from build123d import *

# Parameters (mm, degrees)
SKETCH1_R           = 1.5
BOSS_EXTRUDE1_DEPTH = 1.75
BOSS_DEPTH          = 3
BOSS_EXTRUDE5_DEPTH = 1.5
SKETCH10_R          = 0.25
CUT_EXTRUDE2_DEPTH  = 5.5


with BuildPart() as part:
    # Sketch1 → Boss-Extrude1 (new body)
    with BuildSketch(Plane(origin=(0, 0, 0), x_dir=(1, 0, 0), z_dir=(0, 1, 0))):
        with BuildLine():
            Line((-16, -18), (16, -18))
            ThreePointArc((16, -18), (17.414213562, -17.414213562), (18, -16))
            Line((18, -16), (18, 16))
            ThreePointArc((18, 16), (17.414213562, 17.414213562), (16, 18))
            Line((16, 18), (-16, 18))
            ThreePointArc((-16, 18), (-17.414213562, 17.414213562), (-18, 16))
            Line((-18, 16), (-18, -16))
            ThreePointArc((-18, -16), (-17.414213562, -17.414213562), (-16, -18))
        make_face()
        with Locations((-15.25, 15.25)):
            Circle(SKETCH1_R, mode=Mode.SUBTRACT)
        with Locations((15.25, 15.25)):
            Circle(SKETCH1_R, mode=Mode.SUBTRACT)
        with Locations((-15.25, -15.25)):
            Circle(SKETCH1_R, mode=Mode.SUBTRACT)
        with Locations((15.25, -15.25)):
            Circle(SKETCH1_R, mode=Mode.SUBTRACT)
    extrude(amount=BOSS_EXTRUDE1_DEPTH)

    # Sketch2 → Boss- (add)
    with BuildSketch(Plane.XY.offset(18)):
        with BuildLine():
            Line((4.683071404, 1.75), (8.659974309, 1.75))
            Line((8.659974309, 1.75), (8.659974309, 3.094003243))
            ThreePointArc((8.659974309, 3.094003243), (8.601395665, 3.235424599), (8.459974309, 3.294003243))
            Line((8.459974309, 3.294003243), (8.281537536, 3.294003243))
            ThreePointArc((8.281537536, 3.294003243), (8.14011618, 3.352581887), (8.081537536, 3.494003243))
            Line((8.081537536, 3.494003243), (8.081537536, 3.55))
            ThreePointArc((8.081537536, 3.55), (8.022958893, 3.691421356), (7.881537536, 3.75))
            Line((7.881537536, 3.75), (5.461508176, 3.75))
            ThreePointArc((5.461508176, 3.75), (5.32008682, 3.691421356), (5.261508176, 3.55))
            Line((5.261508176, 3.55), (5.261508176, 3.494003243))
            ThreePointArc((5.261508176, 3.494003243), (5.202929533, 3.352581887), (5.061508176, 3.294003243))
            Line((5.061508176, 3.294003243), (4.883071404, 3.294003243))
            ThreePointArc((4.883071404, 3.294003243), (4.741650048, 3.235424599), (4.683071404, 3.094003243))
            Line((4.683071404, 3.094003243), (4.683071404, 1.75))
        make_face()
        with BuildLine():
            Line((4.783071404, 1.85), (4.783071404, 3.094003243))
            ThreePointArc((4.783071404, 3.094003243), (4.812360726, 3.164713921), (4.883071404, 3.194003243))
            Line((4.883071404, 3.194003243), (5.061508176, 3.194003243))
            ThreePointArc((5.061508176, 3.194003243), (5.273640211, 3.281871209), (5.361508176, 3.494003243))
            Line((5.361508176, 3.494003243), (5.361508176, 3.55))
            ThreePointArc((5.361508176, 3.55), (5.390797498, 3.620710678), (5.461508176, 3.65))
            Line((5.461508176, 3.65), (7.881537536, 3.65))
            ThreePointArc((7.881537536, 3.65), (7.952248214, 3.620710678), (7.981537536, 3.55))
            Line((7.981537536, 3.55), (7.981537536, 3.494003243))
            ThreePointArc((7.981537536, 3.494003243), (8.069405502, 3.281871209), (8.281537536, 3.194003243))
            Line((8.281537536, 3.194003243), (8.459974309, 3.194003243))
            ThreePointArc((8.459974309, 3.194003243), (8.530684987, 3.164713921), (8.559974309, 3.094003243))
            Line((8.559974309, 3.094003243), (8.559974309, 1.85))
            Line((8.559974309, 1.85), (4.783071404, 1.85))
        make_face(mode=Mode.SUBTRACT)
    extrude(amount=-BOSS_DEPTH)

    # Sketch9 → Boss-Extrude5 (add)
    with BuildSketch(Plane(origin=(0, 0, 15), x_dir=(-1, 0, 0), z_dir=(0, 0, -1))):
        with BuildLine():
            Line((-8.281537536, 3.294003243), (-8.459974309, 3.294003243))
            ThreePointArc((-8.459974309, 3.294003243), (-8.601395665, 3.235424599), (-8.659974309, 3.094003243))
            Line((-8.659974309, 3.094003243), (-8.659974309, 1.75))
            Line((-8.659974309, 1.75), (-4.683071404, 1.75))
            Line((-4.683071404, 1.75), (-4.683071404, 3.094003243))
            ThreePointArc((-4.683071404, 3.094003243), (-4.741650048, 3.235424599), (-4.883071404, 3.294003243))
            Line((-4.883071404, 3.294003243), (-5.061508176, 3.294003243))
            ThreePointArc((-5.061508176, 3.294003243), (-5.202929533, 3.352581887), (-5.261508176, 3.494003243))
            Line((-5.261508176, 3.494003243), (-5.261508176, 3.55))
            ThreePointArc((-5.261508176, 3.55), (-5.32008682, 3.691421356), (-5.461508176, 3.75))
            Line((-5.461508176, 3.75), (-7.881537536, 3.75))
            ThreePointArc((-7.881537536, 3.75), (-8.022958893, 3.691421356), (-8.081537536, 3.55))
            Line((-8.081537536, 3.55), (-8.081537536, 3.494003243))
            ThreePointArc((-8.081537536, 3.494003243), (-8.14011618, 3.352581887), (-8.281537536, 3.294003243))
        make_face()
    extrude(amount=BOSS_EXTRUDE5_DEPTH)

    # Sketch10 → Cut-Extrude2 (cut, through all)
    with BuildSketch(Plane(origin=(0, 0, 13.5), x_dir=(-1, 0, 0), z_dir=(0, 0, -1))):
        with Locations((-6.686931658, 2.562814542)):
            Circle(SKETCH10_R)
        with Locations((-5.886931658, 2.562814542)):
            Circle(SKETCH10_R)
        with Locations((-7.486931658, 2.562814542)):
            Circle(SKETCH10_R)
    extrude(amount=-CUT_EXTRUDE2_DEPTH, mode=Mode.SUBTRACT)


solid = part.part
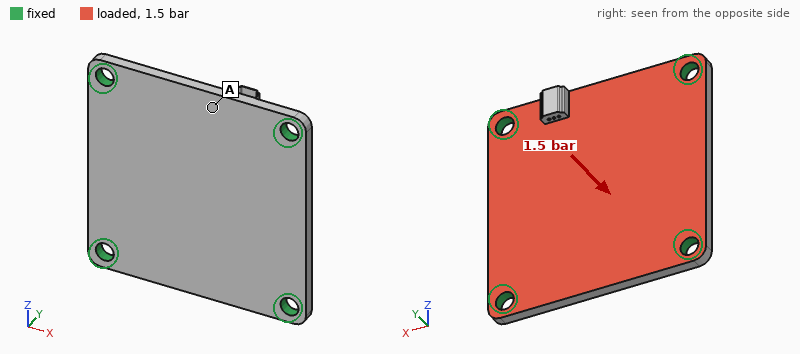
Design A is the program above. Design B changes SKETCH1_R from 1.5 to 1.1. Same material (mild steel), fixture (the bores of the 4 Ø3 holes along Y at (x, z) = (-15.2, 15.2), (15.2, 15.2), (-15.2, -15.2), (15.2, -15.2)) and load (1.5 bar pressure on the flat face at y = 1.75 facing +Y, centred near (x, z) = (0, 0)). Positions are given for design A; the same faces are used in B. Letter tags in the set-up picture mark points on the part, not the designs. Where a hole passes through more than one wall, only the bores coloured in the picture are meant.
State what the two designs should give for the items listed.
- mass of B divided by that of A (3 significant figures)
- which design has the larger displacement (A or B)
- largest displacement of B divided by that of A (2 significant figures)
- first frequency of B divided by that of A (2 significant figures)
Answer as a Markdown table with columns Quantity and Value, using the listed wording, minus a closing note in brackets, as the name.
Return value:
| Quantity | Value |
|---|---|
| mass of B divided by that of A | 1.01 |
| which design has the larger displacement | B |
| largest displacement of B divided by that of A | 1.1 |
| first frequency of B divided by that of A | 0.94 |
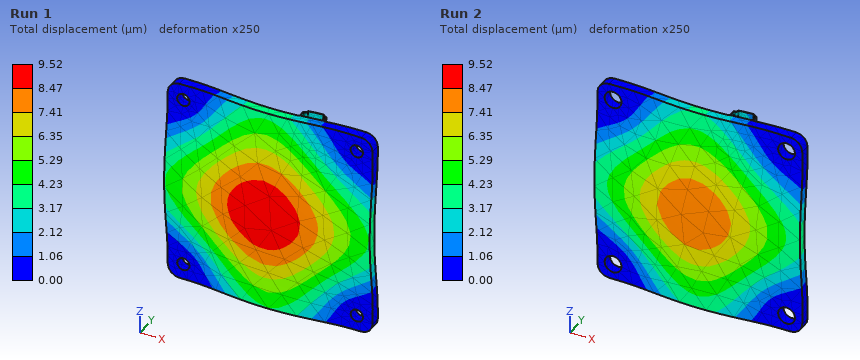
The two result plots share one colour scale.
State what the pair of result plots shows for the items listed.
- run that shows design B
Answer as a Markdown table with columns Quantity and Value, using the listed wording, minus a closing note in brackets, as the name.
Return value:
| Quantity | Value |
|---|---|
| run that shows design B | Run 1 |
